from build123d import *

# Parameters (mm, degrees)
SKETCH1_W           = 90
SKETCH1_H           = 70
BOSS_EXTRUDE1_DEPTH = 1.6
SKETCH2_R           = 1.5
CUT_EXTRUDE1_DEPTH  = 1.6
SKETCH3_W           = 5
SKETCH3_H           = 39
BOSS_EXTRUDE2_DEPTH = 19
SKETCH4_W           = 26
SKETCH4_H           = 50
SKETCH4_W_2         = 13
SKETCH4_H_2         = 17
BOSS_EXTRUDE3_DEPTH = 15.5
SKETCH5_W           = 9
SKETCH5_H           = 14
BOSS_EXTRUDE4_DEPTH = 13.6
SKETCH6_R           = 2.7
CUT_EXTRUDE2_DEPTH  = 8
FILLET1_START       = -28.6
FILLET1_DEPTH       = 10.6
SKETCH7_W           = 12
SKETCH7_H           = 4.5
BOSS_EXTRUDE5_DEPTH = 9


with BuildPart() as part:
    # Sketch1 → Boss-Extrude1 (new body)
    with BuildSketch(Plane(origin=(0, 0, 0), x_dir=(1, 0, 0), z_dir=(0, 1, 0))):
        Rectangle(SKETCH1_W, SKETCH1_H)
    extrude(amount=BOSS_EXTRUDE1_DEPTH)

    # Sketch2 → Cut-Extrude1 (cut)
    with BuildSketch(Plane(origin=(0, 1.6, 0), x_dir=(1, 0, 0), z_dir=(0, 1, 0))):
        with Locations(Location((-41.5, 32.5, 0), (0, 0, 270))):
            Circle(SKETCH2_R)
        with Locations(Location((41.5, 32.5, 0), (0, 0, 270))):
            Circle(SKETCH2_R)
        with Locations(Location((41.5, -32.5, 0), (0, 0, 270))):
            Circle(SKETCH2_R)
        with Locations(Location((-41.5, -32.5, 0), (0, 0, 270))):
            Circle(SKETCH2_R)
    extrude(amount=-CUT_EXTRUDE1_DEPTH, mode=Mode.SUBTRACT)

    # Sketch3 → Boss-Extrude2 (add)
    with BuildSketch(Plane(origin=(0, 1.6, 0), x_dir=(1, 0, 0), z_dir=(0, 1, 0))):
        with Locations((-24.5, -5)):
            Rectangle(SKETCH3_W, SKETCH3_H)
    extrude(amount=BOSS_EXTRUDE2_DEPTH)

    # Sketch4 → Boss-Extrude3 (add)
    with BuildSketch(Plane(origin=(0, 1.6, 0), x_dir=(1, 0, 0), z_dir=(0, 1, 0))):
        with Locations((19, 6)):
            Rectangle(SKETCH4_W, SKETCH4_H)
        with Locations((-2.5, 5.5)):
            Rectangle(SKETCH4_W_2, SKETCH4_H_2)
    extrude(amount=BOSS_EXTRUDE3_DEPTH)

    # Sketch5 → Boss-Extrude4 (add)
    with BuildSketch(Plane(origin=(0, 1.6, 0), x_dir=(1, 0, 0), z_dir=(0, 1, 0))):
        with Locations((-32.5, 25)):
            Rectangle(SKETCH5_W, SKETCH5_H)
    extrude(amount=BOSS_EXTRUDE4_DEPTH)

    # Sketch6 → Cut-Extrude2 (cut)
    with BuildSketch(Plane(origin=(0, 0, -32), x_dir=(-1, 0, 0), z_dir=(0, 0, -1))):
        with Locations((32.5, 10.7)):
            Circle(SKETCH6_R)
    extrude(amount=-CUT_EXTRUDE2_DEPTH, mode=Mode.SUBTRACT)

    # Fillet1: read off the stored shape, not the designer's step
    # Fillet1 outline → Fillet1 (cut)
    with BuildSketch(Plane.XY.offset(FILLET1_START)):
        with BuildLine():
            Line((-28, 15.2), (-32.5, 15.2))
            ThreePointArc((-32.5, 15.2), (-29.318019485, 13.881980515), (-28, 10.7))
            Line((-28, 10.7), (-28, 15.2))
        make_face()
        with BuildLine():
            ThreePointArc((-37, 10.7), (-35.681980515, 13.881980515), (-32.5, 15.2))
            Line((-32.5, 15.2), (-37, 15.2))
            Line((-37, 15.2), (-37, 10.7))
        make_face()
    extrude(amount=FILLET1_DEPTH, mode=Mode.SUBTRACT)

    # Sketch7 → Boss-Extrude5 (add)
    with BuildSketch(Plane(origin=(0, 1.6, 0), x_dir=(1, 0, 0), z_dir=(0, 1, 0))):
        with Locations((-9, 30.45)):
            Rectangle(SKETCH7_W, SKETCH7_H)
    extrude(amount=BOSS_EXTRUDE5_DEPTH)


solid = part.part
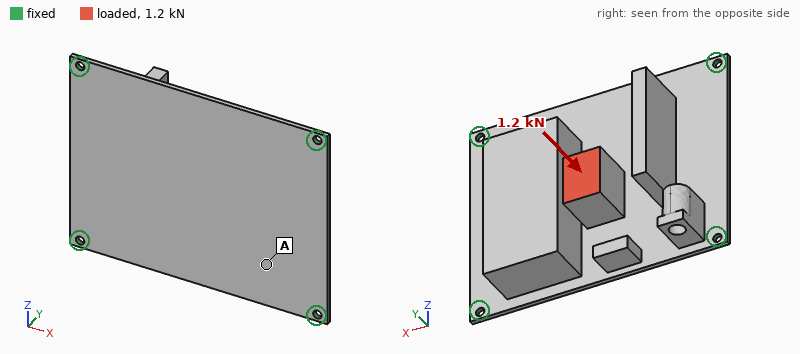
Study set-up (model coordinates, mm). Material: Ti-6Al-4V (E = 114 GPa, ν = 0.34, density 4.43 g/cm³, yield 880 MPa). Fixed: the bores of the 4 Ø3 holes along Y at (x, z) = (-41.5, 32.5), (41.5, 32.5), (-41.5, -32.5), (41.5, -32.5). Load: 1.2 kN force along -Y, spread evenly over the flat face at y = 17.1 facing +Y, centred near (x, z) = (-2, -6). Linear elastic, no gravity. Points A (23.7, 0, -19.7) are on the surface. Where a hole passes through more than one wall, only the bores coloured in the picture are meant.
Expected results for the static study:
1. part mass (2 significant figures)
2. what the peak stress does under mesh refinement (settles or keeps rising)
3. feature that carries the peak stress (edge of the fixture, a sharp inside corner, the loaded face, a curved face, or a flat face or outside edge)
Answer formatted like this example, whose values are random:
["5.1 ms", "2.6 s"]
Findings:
["170 g", "keeps rising", "edge of the fixture"]
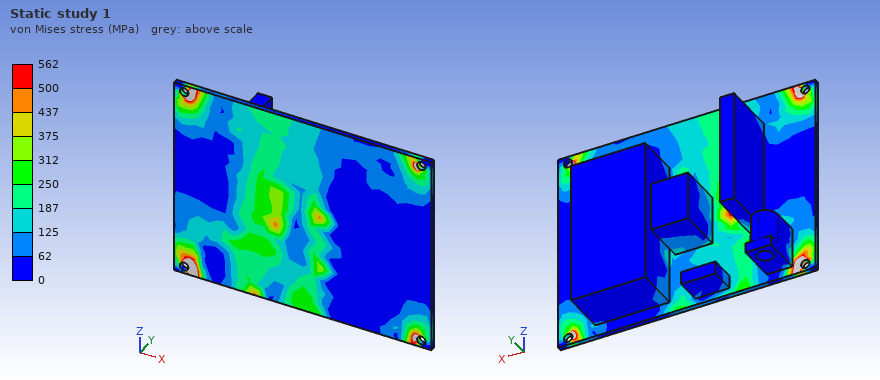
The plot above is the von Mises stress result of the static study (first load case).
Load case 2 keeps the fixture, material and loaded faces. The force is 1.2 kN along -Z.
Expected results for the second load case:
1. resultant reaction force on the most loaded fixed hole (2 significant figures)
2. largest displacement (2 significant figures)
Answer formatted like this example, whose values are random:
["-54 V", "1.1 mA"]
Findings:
["560 N", "0.18 mm"]
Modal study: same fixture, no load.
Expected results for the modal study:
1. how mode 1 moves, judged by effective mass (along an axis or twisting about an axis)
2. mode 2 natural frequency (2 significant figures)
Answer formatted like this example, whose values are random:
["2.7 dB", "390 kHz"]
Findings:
["along Y", "1500 Hz"]
